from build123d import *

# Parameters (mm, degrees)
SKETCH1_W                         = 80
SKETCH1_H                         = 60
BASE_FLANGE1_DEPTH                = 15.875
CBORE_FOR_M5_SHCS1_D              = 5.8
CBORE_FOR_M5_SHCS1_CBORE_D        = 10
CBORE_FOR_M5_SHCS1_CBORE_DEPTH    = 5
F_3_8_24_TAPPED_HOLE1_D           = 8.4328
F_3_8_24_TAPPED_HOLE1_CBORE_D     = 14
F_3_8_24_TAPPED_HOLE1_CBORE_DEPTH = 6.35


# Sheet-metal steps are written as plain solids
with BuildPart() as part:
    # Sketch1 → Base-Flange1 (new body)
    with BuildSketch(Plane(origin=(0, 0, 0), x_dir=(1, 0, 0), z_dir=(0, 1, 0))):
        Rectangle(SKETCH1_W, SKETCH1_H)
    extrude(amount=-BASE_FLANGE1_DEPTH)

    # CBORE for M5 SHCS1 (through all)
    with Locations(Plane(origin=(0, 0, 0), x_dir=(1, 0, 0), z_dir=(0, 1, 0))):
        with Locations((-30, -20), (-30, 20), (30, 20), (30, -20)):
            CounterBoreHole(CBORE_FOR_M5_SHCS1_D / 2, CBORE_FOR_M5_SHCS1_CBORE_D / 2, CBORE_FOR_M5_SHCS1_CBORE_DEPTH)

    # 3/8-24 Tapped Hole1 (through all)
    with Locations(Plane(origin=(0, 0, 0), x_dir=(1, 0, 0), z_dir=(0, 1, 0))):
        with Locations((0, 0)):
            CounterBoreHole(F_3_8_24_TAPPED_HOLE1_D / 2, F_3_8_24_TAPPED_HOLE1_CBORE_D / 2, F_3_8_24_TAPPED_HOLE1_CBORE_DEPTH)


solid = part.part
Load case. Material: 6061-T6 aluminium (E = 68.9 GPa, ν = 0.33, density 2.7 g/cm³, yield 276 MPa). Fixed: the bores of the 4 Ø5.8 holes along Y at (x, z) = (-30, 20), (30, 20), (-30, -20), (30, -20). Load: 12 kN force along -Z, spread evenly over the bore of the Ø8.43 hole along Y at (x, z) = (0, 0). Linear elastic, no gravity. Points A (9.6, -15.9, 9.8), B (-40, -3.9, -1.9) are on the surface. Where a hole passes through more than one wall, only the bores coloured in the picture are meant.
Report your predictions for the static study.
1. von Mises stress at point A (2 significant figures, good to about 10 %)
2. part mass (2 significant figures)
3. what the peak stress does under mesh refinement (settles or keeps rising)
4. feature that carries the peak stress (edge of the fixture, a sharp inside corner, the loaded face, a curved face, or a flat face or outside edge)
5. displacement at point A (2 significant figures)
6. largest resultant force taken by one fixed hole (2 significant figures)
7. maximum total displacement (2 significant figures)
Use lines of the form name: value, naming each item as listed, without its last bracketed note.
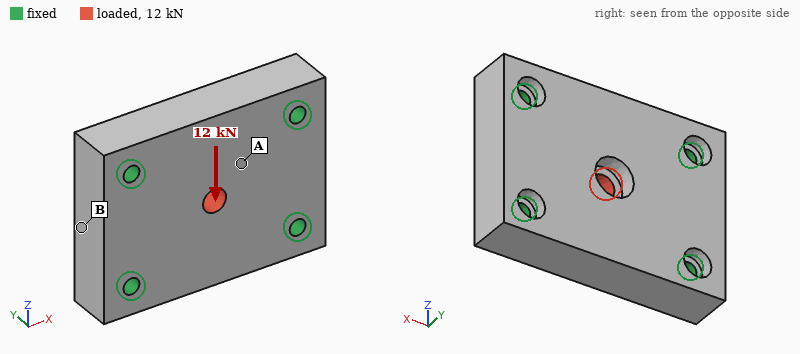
von Mises stress at point A: 24 MPa
part mass: 190 g
what the peak stress does under mesh refinement: keeps rising
feature that carries the peak stress: a sharp inside corner
displacement at point A: 8.8 µm
largest resultant force taken by one fixed hole: 3.4 kN
maximum total displacement: 15 µm
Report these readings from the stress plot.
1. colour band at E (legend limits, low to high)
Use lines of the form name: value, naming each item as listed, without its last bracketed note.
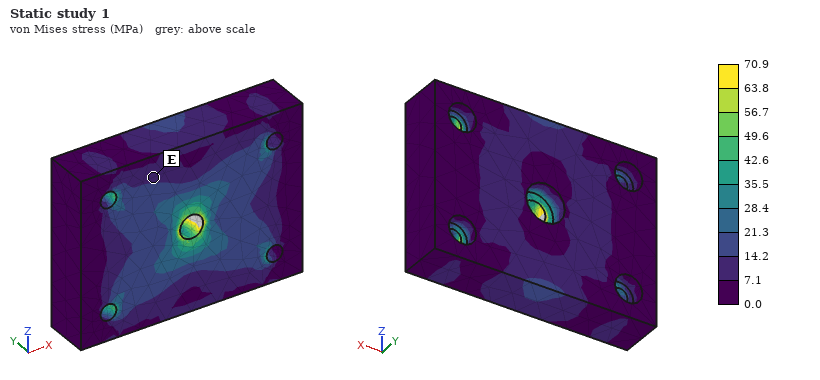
colour band at E: 7.1 to 14.2 MPa
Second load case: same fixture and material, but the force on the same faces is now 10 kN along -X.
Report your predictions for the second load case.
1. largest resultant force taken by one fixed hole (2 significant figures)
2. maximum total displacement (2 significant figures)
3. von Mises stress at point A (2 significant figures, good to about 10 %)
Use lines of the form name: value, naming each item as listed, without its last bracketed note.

largest resultant force taken by one fixed hole: 2.6 kN
maximum total displacement: 9.4 µm
von Mises stress at point A: 16 MPa
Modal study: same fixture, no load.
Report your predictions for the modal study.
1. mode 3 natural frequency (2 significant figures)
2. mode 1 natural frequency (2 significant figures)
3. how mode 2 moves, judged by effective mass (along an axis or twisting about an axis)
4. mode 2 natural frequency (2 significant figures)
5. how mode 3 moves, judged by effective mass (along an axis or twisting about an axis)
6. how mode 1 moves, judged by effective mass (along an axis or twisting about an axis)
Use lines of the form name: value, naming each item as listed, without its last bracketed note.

mode 3 natural frequency: 21 kHz
mode 1 natural frequency: 13 kHz
how mode 2 moves, judged by effective mass: twisting about X
mode 2 natural frequency: 16 kHz
how mode 3 moves, judged by effective mass: along Z
how mode 1 moves, judged by effective mass: along Y
